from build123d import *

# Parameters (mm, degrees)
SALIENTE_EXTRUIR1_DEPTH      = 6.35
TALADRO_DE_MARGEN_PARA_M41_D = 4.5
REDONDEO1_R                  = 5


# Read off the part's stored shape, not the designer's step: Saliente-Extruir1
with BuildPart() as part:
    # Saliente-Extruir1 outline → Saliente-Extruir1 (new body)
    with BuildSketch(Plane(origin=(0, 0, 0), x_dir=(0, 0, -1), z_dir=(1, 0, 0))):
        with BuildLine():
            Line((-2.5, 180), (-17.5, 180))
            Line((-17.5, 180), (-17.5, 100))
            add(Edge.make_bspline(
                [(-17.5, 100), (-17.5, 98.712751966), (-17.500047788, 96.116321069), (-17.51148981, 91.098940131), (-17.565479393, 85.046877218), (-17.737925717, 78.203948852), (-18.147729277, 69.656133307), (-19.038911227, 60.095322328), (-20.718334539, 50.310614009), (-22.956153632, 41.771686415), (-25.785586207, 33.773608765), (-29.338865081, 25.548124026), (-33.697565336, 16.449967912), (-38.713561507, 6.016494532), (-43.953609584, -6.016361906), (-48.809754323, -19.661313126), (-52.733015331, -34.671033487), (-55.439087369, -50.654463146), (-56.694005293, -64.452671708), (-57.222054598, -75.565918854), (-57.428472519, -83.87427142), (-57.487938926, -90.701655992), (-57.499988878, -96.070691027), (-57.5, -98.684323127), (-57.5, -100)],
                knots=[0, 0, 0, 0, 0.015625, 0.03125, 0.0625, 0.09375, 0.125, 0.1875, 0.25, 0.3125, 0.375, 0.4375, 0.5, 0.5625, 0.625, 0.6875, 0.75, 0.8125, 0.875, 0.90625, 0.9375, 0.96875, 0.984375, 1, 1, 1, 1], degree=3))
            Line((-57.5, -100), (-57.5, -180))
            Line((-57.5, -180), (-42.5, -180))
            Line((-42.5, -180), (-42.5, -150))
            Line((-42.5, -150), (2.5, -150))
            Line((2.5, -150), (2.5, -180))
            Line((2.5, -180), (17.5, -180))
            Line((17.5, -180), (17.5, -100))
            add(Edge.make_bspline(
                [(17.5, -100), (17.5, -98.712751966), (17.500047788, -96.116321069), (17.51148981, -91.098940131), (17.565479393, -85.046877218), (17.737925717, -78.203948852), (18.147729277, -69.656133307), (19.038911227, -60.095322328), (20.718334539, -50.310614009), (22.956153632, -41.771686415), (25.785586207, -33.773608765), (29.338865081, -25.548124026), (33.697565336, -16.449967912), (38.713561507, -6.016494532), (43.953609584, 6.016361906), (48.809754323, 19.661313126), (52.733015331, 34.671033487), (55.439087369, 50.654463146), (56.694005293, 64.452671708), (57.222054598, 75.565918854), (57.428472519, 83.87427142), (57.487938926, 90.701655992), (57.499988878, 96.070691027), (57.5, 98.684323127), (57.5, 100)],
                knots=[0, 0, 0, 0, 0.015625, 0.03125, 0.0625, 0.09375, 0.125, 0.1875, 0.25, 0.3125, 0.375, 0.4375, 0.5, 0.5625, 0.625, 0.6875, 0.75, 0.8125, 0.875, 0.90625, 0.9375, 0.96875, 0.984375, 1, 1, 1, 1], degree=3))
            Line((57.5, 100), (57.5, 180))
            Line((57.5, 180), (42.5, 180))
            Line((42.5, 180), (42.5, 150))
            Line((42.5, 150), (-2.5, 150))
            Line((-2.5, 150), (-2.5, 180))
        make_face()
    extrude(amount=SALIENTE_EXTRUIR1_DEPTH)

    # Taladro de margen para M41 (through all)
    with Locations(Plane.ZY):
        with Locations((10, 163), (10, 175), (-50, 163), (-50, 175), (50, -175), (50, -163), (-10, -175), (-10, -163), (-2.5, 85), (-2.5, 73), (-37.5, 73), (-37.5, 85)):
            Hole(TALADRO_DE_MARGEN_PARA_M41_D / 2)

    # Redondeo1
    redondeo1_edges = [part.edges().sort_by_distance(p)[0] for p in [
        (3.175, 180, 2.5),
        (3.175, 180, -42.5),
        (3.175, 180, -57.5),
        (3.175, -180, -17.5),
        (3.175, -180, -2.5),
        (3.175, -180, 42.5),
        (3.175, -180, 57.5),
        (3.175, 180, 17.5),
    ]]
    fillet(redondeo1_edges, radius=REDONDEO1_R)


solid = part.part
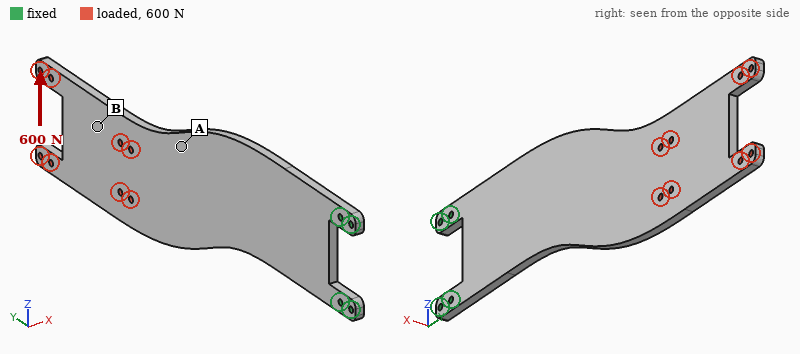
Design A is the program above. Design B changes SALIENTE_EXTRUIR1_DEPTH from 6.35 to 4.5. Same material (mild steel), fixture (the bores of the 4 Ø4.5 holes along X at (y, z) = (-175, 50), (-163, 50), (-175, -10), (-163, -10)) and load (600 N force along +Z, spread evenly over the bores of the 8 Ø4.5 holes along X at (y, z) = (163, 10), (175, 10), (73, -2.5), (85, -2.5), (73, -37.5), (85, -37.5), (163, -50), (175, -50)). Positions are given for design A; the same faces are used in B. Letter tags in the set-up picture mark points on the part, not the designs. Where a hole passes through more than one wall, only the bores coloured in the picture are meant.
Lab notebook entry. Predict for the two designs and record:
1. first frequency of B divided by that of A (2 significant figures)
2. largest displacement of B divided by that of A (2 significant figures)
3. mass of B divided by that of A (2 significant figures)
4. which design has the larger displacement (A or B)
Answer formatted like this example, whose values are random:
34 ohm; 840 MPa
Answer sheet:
0.71; 1.4; 0.71; B
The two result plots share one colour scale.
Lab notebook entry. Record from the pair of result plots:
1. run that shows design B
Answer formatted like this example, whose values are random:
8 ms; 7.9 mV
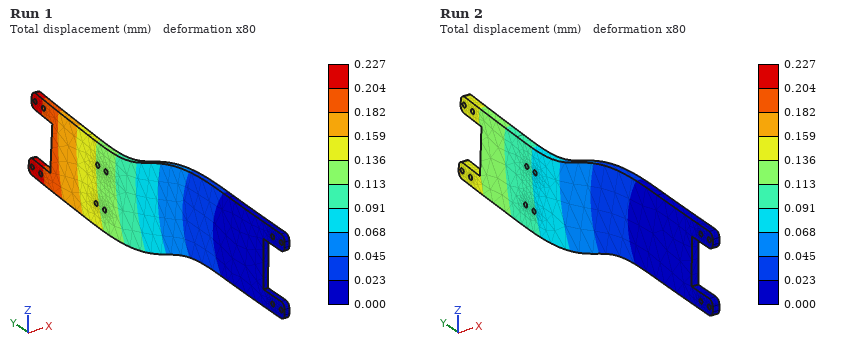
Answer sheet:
Run 1
